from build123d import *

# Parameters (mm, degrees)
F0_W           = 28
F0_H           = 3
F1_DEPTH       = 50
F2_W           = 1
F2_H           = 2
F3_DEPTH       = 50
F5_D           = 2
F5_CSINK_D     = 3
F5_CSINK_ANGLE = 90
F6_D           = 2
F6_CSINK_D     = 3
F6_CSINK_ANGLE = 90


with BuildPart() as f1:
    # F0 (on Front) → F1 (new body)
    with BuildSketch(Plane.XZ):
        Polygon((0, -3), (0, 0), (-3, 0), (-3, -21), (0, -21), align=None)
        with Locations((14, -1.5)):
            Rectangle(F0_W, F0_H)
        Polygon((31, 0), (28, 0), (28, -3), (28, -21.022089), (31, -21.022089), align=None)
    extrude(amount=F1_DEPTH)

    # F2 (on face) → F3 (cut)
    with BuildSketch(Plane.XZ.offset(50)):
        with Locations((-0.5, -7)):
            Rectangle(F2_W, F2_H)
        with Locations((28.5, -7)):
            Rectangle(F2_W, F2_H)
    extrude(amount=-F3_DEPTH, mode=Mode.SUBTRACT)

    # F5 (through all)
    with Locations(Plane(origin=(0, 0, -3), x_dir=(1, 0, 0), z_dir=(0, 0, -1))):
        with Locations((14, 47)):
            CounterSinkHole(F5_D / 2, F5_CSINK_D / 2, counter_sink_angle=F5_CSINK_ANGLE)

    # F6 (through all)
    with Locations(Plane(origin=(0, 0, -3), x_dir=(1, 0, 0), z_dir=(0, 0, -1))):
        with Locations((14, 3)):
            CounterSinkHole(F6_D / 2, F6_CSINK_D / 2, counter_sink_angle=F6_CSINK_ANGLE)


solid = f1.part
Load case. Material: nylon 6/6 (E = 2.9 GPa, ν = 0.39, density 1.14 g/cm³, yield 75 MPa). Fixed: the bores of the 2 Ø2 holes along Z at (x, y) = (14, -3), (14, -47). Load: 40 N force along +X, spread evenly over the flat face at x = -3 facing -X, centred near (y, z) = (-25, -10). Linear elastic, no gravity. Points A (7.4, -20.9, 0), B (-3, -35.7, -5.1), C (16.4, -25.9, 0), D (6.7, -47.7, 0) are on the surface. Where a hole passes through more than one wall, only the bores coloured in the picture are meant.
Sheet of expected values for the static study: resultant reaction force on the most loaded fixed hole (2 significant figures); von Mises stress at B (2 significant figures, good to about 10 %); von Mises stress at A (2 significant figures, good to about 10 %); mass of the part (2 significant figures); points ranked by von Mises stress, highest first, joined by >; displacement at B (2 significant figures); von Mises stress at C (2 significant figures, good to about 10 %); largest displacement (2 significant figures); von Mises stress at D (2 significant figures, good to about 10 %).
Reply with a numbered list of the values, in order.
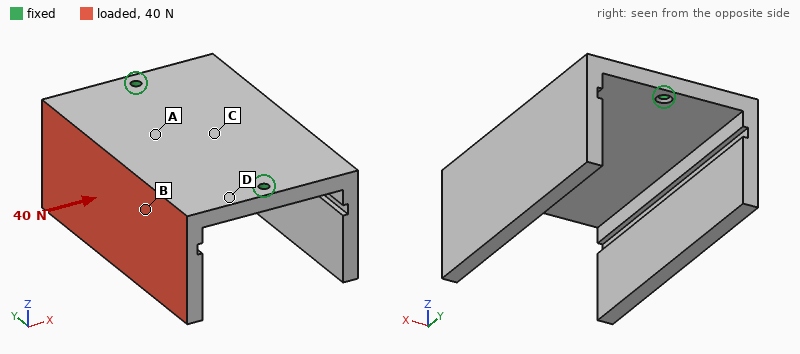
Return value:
1. 20 N
2. 4.3 MPa
3. 3.2 MPa
4. 12 g
5. D > B > A > C
6. 0.28 mm
7. 1.6 MPa
8. 0.62 mm
9. 5.7 MPa
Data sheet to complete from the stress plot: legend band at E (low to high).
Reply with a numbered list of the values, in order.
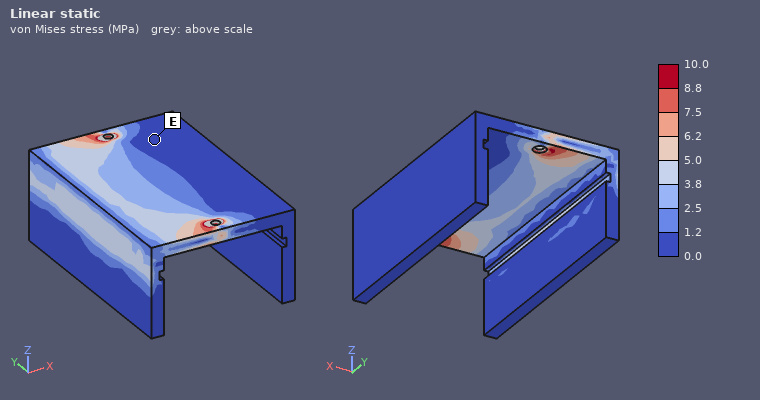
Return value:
1. 0.0 to 1.2 MPa
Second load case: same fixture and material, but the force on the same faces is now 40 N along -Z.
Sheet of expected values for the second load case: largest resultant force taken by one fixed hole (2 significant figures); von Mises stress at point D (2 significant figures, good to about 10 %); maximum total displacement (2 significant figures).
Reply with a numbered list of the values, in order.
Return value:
1. 20 N
2. 8.3 MPa
3. 0.73 mm
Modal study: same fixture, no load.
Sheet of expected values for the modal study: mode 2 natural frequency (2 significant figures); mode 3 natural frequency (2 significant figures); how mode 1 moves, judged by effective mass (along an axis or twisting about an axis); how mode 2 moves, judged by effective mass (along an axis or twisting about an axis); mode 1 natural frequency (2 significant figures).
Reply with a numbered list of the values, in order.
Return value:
1. 850 Hz
2. 1200 Hz
3. along X
4. along Z
5. 550 Hz
